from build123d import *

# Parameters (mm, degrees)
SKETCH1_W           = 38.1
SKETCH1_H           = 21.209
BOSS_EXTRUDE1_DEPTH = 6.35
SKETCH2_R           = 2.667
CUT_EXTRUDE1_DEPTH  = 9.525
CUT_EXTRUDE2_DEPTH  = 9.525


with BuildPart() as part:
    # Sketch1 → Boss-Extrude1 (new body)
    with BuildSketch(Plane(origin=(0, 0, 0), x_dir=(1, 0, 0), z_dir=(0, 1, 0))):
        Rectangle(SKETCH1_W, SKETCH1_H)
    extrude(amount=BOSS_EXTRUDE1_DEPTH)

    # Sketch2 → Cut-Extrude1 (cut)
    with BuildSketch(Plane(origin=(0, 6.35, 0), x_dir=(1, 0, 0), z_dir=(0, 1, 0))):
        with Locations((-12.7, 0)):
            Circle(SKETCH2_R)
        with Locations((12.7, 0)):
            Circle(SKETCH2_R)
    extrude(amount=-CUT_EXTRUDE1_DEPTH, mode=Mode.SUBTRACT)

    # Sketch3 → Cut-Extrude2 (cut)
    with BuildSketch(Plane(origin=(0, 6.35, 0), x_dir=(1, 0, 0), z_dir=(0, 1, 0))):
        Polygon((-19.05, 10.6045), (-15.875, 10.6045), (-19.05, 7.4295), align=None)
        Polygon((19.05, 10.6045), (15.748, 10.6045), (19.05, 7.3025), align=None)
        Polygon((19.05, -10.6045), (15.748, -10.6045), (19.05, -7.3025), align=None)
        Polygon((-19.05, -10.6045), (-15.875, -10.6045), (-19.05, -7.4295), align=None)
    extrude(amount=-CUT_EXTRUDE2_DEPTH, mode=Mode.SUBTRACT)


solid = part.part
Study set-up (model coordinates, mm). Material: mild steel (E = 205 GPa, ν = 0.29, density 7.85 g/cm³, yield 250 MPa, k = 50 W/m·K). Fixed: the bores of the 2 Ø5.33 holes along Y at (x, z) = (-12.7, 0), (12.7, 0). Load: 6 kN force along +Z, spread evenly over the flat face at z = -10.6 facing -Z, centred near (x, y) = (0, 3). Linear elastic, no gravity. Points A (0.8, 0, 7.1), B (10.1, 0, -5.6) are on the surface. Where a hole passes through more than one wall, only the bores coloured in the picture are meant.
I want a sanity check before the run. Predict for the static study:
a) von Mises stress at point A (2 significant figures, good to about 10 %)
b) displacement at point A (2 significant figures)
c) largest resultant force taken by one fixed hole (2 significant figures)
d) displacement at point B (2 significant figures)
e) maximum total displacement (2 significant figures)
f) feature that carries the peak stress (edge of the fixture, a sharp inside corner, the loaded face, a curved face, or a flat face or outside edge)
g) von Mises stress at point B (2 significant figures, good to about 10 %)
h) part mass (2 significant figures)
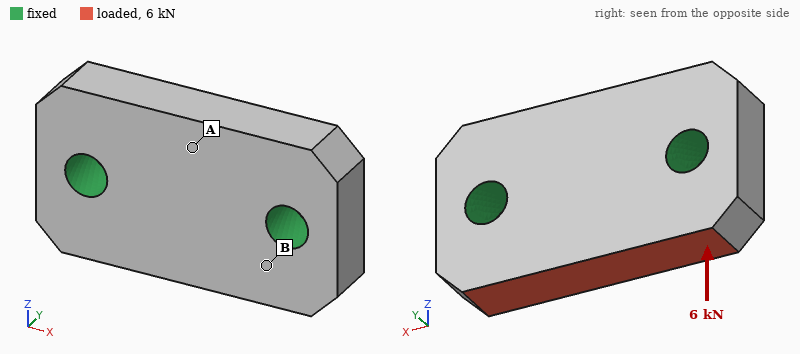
12 MPa
1.5 µm
3.1 kN
1.0 µm
2.9 µm
edge of the fixture
40 MPa
37 g
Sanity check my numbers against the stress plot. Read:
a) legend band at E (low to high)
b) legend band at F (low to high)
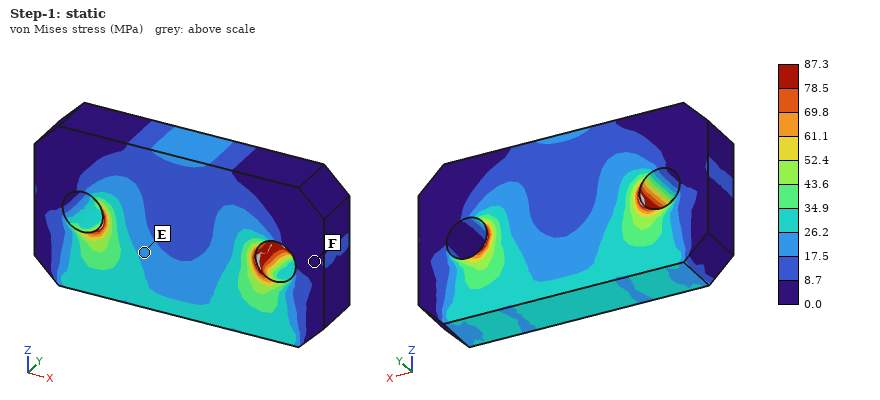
17.5 to 26.2 MPa
0.0 to 8.7 MPa
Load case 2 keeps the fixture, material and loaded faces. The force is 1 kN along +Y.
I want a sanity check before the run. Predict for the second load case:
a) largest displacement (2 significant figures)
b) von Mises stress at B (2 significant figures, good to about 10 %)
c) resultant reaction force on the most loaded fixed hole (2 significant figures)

4.7 µm
27 MPa
500 N
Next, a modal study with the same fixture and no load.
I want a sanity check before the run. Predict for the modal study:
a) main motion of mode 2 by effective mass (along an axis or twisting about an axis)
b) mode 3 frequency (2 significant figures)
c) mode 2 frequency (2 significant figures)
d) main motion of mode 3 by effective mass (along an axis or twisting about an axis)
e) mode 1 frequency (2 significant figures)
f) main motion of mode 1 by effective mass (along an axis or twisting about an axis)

along Y
52 kHz
35 kHz
along Z
33 kHz
twisting about X
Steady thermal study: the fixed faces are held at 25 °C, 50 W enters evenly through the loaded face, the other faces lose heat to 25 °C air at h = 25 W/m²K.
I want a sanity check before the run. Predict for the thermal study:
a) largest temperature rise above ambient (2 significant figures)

58 K
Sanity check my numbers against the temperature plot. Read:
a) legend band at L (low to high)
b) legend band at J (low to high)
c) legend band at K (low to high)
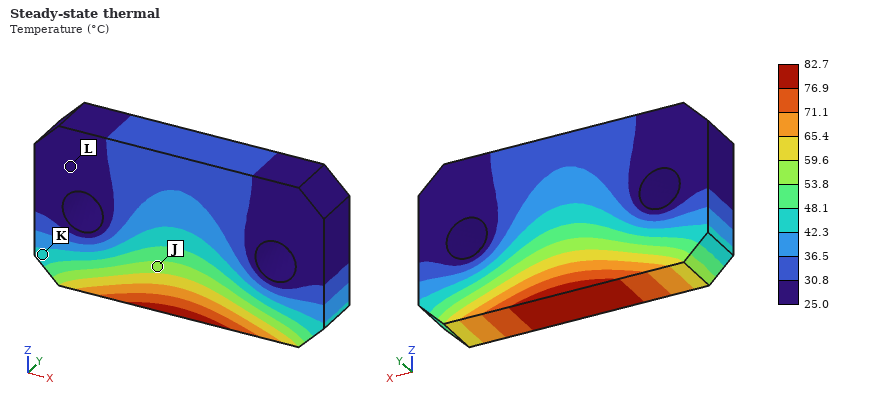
25.0 to 30.8 °C
53.8 to 59.6 °C
42.3 to 48.1 °C
